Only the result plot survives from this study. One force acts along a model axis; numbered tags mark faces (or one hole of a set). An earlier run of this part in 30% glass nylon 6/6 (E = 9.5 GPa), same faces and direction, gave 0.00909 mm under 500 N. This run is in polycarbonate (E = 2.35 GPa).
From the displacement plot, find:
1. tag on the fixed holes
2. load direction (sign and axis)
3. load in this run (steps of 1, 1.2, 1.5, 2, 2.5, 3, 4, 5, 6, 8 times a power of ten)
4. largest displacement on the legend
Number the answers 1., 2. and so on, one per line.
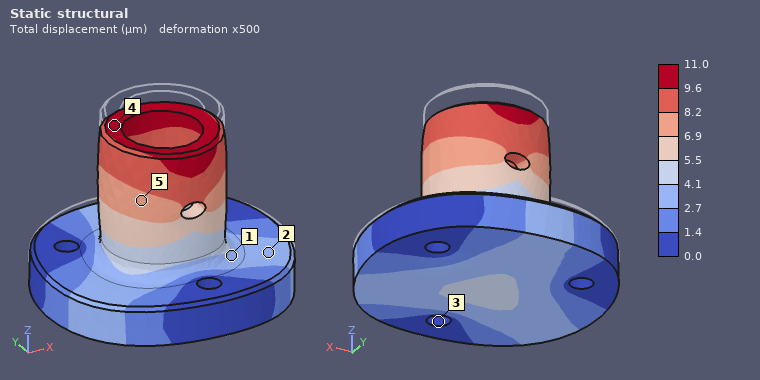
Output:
1. 3
2. -Z
3. 150 N
4. 11.0 µm
